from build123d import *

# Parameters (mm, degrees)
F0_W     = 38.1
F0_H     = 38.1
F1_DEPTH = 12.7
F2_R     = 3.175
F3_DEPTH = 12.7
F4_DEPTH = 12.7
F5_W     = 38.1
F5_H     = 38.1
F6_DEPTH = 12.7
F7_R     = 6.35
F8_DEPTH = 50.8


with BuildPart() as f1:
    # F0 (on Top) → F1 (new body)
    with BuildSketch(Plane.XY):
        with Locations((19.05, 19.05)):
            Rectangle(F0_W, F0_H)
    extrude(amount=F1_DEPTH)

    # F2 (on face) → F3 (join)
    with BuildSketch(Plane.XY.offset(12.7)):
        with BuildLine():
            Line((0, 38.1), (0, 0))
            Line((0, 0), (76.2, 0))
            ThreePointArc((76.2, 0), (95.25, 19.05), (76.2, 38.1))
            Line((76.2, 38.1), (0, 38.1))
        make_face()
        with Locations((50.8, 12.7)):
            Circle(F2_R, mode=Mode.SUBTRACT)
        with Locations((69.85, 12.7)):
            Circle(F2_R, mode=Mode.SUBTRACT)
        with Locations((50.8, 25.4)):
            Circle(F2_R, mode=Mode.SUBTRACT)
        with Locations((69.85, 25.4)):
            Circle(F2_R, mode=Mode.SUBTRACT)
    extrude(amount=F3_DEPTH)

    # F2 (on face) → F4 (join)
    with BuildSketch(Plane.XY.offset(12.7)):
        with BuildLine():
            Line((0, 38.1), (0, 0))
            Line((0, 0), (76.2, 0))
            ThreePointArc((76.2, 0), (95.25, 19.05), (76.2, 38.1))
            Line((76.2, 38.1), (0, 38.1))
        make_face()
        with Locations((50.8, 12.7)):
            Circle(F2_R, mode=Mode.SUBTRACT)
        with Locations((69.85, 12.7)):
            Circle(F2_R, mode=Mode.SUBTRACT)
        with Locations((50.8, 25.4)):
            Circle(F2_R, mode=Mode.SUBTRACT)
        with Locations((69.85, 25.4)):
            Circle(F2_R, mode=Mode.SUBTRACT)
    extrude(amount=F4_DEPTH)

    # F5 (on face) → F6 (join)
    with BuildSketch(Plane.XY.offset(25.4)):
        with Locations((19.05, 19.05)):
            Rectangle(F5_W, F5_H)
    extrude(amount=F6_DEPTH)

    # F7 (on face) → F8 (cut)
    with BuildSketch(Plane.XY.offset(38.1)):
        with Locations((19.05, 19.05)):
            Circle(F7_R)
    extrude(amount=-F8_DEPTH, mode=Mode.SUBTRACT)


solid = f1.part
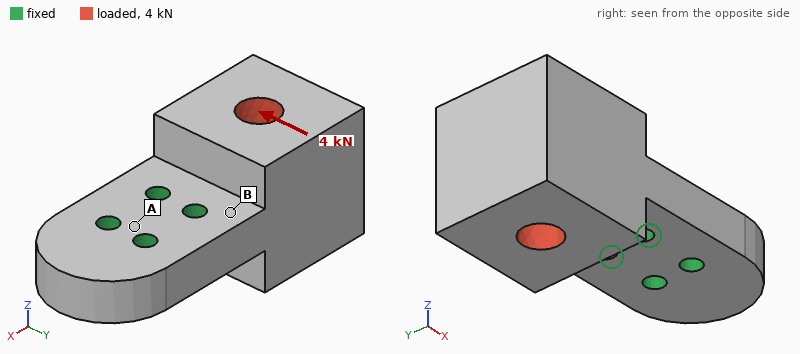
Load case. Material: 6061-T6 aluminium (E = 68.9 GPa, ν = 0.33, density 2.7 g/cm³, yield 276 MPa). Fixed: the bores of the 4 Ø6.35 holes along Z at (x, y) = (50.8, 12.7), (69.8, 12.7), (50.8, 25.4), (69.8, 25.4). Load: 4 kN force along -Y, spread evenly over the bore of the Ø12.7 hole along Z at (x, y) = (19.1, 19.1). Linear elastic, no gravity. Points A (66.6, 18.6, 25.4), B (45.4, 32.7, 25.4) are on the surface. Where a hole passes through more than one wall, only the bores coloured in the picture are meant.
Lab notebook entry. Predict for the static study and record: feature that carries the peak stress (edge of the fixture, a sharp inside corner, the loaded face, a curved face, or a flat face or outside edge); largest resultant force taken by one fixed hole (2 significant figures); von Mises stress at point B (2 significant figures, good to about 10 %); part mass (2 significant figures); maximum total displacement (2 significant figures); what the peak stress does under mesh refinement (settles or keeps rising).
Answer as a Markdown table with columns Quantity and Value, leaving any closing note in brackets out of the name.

| Quantity | Value |
|---|---|
| feature that carries the peak stress | edge of the fixture |
| largest resultant force taken by one fixed hole | 5.1 kN |
| von Mises stress at point B | 22 MPa |
| part mass | 200 g |
| maximum total displacement | 40 µm |
| what the peak stress does under mesh refinement | keeps rising |
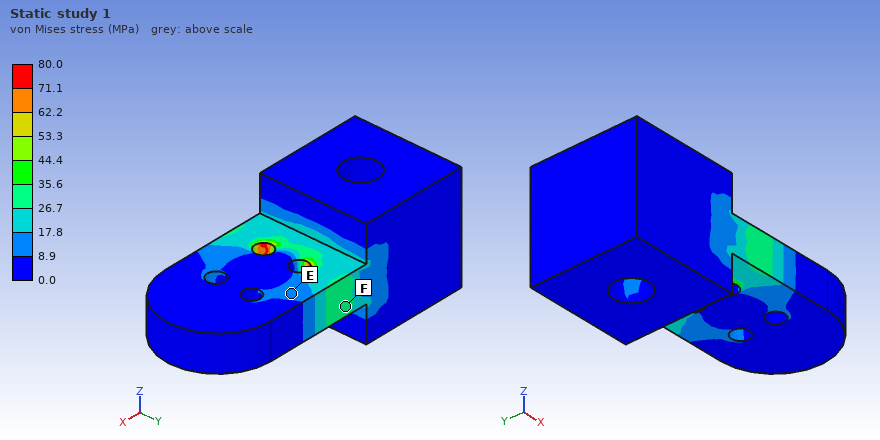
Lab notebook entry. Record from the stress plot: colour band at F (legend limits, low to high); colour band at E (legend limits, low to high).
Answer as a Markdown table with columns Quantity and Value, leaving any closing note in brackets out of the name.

| Quantity | Value |
|---|---|
| colour band at F | 26.7 to 35.6 MPa |
| colour band at E | 8.9 to 17.8 MPa |
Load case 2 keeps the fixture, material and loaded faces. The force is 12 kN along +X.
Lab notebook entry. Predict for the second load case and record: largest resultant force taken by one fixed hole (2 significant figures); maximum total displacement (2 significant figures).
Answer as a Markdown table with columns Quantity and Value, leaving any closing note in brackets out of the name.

| Quantity | Value |
|---|---|
| largest resultant force taken by one fixed hole | 5.4 kN |
| maximum total displacement | 12 µm |
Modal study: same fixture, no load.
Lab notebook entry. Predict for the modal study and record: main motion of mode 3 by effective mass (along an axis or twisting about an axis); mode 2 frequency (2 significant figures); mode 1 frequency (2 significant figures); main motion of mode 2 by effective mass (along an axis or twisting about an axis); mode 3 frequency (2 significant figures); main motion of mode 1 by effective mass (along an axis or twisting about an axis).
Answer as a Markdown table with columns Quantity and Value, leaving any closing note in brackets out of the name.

| Quantity | Value |
|---|---|
| main motion of mode 3 by effective mass | twisting about X |
| mode 2 frequency | 5000 Hz |
| mode 1 frequency | 2500 Hz |
| main motion of mode 2 by effective mass | along Y |
| mode 3 frequency | 6500 Hz |
| main motion of mode 1 by effective mass | along Z |
